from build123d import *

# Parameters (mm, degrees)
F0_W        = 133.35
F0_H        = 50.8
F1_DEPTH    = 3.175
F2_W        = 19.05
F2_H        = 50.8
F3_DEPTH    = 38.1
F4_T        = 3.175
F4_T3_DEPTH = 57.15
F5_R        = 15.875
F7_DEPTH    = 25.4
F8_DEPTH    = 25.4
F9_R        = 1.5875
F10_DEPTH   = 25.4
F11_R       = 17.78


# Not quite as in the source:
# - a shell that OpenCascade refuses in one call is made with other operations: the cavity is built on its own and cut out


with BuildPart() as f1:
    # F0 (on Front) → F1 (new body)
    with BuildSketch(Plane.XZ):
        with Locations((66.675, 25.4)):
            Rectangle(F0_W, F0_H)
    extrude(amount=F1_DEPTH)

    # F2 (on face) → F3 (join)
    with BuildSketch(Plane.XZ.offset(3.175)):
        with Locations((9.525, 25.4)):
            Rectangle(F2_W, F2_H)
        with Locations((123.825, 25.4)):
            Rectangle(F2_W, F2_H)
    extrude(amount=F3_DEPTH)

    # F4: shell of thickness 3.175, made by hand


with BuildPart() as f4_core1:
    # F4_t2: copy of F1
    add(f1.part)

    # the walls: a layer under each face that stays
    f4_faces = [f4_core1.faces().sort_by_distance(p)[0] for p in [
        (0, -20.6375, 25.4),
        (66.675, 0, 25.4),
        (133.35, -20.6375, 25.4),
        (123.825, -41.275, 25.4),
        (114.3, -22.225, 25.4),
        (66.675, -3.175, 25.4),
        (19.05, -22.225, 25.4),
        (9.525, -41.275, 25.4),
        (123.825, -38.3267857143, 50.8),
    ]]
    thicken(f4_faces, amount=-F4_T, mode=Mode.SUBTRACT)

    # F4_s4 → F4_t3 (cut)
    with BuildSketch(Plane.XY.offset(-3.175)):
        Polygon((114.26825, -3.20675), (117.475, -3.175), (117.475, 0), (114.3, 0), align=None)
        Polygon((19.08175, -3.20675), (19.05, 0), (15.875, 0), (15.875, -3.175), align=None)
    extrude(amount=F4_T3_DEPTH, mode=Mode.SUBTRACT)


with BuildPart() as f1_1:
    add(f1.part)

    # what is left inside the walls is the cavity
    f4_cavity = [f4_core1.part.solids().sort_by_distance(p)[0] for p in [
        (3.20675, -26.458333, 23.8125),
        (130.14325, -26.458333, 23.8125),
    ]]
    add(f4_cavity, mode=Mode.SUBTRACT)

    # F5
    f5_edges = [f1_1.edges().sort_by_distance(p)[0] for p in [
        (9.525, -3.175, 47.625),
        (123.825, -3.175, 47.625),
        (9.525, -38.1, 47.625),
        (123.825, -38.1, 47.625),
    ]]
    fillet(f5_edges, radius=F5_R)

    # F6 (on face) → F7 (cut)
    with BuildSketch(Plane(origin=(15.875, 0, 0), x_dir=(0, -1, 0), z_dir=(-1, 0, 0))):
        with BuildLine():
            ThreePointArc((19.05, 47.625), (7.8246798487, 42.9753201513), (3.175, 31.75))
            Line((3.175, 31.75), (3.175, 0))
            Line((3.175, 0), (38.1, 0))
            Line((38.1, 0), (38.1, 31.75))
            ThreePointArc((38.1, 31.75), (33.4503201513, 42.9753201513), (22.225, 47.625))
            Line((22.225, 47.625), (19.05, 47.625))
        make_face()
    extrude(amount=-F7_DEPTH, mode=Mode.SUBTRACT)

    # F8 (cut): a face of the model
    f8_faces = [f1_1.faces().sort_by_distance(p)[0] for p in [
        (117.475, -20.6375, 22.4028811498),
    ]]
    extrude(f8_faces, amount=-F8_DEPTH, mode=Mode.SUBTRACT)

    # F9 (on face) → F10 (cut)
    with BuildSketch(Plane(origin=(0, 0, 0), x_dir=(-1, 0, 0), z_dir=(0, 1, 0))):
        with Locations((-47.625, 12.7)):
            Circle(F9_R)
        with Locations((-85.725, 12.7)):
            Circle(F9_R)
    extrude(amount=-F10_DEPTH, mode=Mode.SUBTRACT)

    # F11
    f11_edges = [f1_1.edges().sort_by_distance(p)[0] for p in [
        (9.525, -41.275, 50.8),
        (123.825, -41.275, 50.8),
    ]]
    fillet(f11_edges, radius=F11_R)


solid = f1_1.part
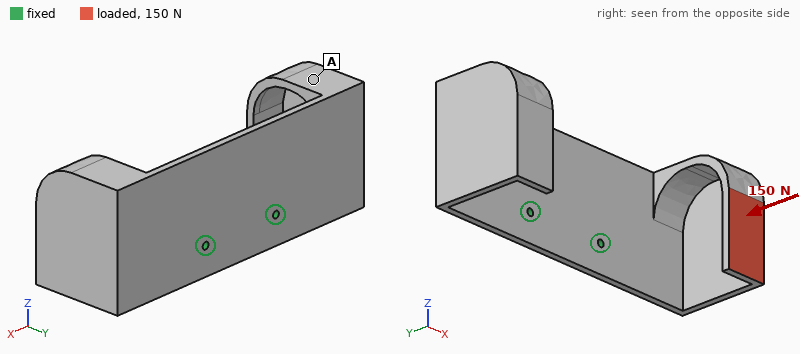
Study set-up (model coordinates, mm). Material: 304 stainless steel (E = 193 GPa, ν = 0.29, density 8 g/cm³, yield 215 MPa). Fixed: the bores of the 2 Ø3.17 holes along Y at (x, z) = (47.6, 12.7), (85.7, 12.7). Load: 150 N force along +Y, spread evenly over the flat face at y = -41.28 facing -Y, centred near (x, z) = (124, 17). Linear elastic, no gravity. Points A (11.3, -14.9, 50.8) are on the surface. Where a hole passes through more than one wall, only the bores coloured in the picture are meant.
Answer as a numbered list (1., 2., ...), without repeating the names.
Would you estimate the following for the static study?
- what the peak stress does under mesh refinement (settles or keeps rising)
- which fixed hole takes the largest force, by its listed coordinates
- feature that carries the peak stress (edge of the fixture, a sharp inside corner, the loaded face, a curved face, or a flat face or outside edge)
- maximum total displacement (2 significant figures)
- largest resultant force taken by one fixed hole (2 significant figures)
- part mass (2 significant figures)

1. keeps rising
2. (85.7, 12.7)
3. edge of the fixture
4. 0.27 mm
5. 220 N
6. 350 g
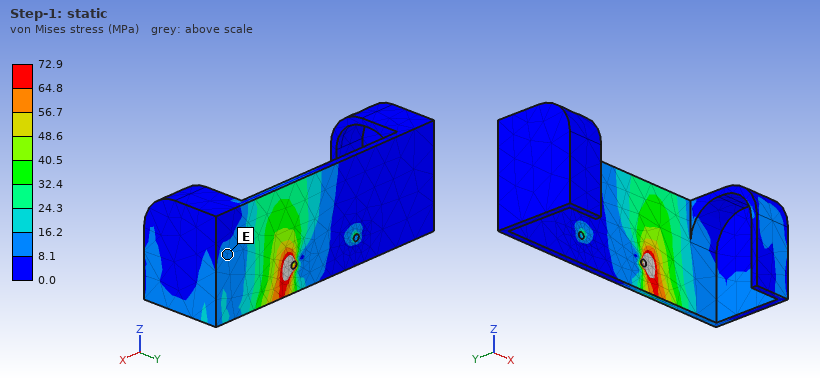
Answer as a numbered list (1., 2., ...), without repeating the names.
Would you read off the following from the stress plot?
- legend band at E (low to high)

1. 8.1 to 16.2 MPa
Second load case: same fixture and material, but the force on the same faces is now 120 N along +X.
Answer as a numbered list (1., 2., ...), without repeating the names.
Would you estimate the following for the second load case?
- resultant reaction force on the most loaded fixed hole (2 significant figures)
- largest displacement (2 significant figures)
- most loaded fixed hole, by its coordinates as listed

1. 110 N
2. 0.39 mm
3. (85.7, 12.7)
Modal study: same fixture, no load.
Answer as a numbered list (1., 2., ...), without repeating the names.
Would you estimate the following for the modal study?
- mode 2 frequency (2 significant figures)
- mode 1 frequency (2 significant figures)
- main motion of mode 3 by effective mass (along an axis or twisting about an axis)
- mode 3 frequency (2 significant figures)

1. 330 Hz
2. 320 Hz
3. along Z
4. 500 Hz
